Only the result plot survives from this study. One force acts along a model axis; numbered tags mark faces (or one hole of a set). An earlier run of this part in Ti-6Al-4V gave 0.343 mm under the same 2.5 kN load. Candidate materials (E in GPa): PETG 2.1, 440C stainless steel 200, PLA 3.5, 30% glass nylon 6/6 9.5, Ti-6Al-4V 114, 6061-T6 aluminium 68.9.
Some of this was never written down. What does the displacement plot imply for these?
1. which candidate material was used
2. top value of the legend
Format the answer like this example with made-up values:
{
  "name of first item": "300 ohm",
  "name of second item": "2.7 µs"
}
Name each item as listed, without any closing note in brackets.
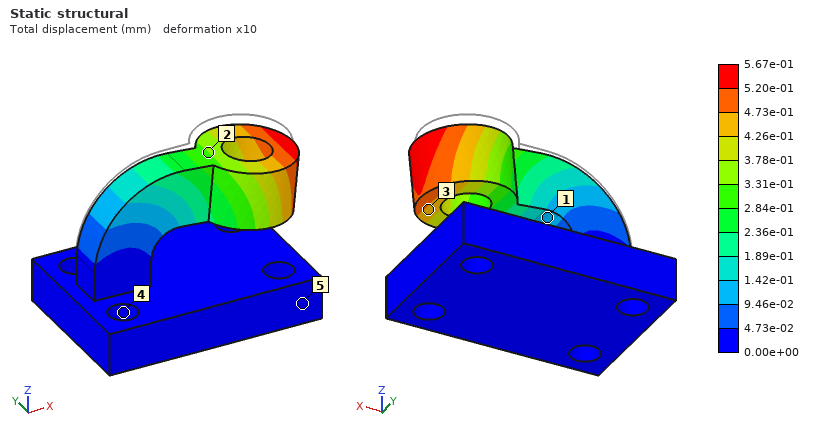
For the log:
{
  "which candidate material was used": "6061-T6 aluminium",
  "top value of the legend": "5.67e-01 mm"
}
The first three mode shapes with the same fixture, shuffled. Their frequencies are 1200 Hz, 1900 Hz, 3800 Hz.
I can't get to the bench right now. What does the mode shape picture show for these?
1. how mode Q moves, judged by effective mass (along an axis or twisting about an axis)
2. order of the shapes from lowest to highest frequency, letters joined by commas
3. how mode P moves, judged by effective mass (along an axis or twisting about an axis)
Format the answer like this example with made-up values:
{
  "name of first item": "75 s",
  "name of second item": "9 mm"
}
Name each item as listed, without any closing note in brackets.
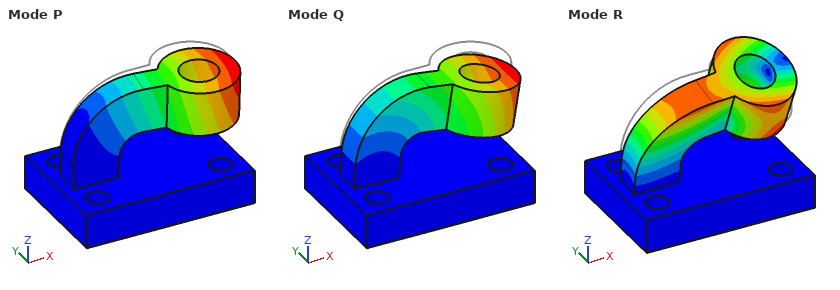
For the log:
{
  "how mode Q moves, judged by effective mass": "along Z",
  "order of the shapes from lowest to highest frequency, letters joined by commas": "P, Q, R",
  "how mode P moves, judged by effective mass": "along Y"
}
